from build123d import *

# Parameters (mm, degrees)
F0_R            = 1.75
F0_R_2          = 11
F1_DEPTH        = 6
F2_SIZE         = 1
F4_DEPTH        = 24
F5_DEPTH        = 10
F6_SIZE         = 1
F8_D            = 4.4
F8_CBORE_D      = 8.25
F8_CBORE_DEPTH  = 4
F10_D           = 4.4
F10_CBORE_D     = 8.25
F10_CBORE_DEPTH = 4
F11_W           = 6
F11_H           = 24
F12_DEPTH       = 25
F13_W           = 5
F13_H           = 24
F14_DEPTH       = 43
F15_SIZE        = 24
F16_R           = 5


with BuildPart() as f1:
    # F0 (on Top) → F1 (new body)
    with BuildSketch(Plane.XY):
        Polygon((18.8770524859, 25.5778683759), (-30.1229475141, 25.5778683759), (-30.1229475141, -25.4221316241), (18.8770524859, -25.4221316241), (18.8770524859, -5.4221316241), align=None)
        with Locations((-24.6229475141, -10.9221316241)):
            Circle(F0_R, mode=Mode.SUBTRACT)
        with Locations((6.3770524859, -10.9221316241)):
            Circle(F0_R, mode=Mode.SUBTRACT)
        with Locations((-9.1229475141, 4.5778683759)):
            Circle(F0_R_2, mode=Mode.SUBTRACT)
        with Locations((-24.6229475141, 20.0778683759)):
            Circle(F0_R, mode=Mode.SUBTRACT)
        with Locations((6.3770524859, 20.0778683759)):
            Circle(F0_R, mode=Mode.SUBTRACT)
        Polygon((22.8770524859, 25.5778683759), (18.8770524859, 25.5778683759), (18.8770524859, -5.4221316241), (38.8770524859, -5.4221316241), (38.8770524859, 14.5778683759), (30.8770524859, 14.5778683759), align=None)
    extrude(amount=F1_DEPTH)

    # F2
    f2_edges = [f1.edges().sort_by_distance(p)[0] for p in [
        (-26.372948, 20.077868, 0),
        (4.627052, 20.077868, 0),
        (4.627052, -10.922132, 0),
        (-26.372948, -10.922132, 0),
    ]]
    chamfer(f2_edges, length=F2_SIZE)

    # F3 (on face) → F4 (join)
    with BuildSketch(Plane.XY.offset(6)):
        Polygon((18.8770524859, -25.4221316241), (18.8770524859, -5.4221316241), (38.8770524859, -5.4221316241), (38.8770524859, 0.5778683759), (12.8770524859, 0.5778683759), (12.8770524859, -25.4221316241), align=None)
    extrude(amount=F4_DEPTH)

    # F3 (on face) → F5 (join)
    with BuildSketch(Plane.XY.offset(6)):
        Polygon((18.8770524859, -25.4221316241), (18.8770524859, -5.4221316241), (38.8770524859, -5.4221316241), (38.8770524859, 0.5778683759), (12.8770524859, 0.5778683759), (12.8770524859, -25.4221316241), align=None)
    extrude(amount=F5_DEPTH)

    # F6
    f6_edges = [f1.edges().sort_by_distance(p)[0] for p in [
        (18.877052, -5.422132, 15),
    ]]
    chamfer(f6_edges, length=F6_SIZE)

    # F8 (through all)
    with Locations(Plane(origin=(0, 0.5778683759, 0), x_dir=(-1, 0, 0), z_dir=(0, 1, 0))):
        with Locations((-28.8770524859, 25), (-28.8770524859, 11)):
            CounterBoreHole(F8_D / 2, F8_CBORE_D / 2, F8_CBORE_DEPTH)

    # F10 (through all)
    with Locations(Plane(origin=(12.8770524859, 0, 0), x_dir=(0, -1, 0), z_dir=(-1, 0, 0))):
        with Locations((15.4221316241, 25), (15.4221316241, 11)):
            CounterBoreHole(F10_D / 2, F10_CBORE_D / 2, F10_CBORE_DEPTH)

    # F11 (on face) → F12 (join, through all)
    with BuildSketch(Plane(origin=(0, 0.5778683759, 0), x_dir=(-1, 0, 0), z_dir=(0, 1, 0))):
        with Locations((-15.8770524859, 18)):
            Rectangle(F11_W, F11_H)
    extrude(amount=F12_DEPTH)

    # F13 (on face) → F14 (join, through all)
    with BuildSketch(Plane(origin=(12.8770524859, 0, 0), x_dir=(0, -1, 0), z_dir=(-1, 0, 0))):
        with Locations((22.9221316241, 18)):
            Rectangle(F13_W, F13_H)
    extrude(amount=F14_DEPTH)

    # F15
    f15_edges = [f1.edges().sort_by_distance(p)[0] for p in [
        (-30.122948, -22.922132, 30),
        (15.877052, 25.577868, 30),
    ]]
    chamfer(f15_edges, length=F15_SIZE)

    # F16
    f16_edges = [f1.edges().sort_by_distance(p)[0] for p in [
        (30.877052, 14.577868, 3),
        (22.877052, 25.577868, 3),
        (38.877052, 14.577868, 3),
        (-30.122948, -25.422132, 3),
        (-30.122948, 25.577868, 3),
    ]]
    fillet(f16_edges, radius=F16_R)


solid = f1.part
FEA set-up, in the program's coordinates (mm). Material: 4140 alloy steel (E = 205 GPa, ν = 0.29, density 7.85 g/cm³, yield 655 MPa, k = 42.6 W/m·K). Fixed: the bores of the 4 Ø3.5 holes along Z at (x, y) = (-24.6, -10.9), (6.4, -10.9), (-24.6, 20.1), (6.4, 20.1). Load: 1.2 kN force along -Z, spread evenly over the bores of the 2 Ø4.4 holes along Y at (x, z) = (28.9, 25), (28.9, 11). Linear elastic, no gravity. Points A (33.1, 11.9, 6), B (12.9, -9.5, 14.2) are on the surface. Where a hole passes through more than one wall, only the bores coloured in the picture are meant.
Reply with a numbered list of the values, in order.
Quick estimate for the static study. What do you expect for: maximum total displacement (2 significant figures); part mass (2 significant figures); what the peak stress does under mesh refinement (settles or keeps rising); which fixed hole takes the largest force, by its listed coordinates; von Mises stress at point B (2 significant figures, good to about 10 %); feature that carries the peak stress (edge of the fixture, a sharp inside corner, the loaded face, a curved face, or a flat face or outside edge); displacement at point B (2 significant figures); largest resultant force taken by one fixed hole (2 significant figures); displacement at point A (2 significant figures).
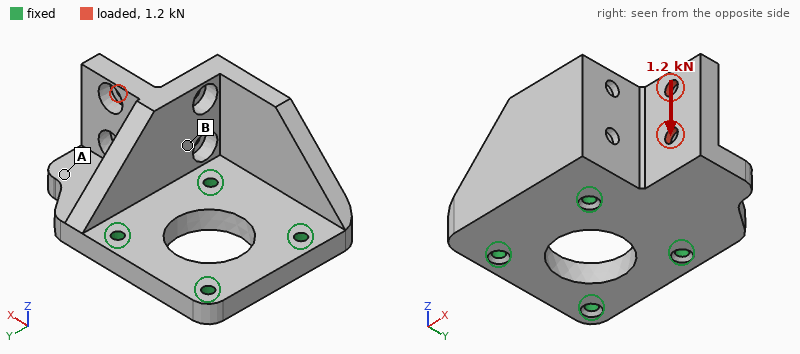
1. 44 µm
2. 210 g
3. keeps rising
4. (6.4, -10.9)
5. 23 MPa
6. edge of the fixture
7. 9.8 µm
8. 1.4 kN
9. 23 µm
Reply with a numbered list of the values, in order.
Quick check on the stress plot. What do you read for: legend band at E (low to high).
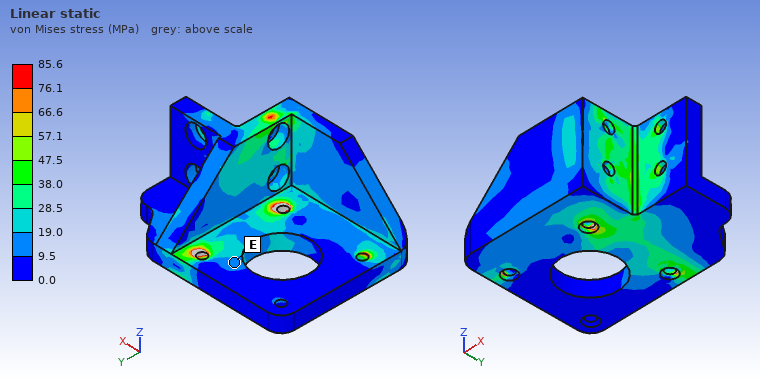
1. 9.5 to 19.0 MPa
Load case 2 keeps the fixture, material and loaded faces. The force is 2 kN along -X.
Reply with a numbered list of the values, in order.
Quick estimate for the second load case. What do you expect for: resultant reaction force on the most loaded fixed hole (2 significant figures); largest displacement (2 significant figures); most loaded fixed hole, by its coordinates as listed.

1. 1.4 kN
2. 54 µm
3. (6.4, -10.9)
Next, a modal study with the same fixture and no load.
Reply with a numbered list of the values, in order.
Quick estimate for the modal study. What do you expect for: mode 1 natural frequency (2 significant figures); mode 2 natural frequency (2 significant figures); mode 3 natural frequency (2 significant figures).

1. 4300 Hz
2. 7200 Hz
3. 11 kHz
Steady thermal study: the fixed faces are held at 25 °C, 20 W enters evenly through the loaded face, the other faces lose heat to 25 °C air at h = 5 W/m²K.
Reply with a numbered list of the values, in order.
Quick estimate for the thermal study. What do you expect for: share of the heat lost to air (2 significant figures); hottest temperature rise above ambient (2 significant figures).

1. 5.4 %
2. 87 K
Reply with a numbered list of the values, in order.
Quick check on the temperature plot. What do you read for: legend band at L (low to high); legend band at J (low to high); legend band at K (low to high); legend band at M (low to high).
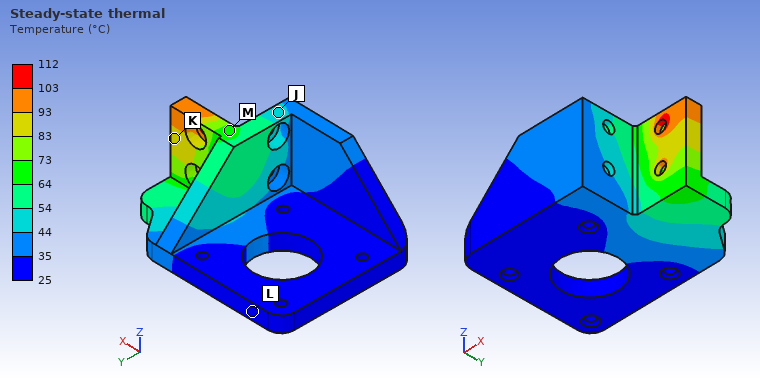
1. 25 to 35 °C
2. 44 to 54 °C
3. 83 to 93 °C
4. 64 to 73 °C
